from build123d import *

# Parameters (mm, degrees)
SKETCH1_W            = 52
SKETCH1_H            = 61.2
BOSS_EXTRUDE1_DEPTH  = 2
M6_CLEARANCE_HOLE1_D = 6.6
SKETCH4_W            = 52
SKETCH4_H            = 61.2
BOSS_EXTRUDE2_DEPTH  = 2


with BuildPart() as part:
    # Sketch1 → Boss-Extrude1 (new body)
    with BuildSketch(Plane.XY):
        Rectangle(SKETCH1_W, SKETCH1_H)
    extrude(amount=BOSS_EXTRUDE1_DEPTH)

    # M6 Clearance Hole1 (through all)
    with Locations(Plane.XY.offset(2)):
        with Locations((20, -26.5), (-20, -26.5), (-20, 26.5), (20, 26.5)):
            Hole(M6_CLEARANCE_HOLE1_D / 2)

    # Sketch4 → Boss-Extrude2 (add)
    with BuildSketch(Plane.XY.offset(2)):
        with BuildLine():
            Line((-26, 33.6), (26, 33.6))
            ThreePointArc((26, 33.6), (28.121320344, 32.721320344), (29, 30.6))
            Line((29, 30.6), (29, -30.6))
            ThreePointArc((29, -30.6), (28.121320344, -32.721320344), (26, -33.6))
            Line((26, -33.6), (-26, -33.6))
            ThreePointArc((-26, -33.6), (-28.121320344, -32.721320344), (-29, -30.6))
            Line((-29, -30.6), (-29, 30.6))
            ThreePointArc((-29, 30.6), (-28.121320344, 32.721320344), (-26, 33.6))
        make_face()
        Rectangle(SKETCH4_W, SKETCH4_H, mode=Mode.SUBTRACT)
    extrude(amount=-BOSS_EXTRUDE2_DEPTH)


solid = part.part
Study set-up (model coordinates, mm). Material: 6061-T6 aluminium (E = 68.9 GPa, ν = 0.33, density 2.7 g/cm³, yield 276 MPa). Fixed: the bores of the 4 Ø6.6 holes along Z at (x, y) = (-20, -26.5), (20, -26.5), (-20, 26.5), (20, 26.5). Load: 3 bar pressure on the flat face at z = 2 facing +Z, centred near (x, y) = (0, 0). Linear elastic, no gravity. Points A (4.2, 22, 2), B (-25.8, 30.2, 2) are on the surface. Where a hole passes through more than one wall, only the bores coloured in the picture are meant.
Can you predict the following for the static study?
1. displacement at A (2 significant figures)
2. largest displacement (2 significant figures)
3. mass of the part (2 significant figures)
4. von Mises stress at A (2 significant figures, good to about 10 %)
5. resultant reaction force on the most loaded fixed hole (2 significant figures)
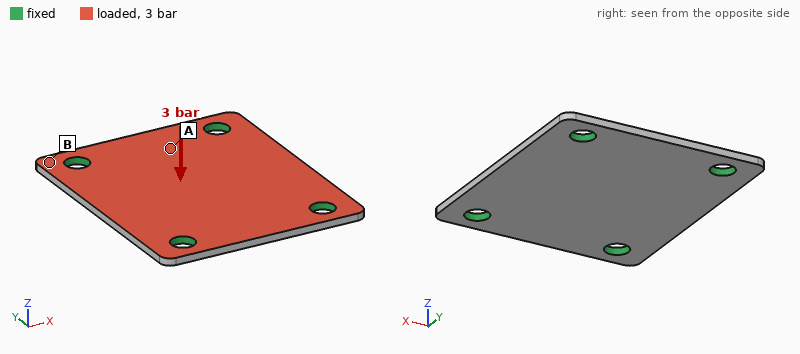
0.051 mm
0.14 mm
20 g
32 MPa
280 N
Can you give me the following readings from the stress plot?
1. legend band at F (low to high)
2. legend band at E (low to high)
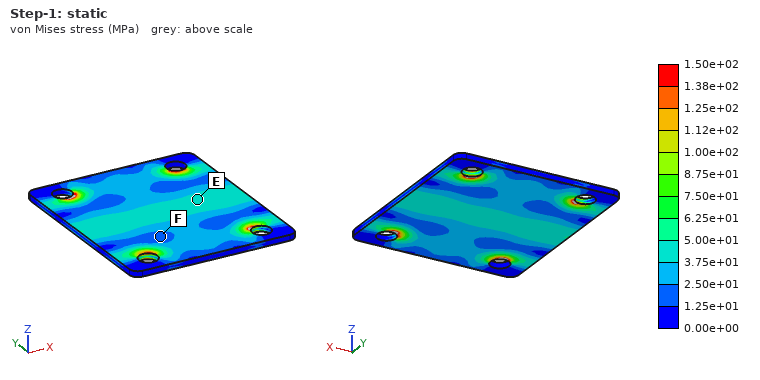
1.25e+01 to 2.50e+01 MPa
3.75e+01 to 5.00e+01 MPa
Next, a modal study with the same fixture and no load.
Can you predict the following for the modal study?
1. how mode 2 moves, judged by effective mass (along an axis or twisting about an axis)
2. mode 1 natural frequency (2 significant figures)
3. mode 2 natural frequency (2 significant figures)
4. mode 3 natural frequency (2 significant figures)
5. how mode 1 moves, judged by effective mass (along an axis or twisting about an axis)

twisting about Y
3800 Hz
4900 Hz
6200 Hz
along Z
